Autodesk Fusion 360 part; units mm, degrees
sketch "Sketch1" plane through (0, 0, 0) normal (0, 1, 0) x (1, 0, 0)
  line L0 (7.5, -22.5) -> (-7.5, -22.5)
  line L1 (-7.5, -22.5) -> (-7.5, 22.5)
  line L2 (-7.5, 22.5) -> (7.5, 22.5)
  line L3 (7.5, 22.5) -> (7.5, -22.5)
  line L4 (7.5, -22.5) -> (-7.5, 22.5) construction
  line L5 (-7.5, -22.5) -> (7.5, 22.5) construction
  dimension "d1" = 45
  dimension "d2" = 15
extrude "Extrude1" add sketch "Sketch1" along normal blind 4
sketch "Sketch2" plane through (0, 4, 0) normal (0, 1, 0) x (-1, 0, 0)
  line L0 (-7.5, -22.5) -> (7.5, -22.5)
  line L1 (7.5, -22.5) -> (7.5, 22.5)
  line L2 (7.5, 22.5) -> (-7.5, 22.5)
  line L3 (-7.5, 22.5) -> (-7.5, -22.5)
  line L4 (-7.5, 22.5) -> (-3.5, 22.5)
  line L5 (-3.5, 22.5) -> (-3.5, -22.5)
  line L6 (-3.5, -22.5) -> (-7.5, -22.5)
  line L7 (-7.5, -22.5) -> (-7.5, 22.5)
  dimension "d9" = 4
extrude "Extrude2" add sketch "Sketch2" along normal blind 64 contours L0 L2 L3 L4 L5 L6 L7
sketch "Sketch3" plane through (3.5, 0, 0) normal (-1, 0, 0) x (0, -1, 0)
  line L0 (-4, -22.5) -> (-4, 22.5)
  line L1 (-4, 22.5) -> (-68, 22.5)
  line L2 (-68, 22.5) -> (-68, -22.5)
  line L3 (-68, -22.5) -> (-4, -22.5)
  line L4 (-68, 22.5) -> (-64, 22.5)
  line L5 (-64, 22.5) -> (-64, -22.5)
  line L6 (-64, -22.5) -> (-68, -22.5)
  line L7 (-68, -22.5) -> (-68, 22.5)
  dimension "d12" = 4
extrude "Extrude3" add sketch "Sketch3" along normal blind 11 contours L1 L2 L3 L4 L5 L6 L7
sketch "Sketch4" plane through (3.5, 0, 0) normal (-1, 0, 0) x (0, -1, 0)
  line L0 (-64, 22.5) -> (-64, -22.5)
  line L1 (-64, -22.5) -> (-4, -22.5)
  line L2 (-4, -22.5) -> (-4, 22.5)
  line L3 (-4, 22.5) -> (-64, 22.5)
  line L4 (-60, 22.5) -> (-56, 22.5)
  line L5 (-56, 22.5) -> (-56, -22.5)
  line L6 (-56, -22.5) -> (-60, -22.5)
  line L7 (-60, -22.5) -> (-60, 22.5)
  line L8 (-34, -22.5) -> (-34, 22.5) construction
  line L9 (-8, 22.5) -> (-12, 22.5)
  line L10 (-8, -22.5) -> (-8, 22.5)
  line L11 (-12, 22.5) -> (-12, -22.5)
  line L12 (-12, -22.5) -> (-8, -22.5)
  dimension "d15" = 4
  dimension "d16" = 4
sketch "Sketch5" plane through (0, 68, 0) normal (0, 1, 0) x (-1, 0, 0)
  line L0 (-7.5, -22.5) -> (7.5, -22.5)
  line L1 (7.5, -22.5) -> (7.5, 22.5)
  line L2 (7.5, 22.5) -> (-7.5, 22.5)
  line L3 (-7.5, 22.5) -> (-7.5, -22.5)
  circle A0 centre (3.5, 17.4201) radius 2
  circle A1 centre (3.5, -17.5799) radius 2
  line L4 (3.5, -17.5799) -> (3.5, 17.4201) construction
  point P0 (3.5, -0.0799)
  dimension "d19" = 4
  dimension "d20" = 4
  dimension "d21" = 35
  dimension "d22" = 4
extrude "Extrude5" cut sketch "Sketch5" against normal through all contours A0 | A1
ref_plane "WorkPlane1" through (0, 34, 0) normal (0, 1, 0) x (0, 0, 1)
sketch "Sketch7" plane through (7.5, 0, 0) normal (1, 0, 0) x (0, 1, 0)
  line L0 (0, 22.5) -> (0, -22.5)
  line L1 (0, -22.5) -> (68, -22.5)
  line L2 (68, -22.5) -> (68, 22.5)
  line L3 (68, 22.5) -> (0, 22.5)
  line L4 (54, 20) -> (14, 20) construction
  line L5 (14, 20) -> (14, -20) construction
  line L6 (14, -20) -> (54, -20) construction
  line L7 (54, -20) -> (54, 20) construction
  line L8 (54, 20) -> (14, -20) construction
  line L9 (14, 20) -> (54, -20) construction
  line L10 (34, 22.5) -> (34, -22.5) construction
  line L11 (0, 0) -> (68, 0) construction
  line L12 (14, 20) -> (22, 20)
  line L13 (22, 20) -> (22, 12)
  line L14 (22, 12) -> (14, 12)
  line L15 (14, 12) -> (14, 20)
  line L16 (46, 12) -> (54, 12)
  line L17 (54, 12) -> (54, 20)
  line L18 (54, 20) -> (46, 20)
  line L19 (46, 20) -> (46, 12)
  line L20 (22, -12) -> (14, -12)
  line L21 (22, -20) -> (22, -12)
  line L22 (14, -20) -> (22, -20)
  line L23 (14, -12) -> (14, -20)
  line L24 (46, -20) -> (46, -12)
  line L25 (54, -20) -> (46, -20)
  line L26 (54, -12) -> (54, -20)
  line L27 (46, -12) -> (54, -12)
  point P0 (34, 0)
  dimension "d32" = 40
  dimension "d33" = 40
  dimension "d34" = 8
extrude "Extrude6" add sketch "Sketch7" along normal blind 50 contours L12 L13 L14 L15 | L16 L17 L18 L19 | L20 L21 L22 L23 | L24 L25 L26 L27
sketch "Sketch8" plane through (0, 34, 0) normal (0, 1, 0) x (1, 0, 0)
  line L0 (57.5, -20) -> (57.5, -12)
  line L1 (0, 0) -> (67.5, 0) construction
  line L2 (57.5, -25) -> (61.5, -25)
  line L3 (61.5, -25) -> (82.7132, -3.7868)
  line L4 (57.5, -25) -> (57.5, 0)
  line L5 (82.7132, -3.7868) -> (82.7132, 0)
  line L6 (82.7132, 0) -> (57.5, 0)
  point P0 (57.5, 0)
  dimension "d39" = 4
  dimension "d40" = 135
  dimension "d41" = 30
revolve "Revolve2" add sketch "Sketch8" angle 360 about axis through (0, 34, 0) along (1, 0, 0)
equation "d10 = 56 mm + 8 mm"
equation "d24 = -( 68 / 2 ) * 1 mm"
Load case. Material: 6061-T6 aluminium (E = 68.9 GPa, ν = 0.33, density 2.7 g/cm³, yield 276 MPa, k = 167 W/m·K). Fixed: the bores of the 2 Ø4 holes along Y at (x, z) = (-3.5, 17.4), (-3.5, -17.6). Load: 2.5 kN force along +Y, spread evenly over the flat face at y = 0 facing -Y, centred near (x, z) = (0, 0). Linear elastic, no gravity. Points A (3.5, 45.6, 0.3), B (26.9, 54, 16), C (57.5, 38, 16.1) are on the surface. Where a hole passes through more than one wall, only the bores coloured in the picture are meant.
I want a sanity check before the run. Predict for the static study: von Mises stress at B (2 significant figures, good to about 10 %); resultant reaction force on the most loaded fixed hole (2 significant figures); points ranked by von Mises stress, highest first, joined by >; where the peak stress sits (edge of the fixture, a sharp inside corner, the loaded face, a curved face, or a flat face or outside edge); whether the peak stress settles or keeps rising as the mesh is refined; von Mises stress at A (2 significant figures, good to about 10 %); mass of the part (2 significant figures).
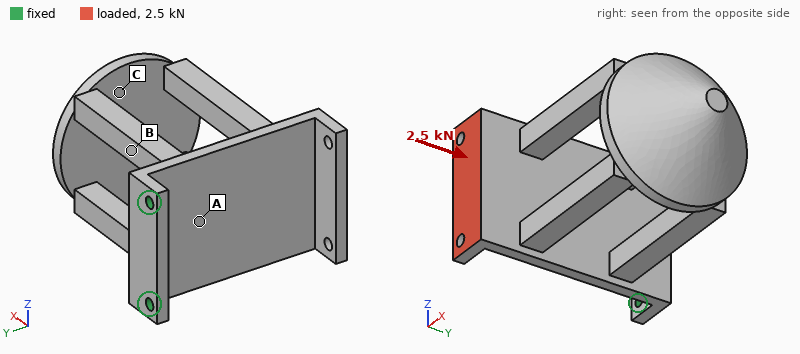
26 MPa
1.3 kN
A > B > C
edge of the fixture
keeps rising
52 MPa
140 g
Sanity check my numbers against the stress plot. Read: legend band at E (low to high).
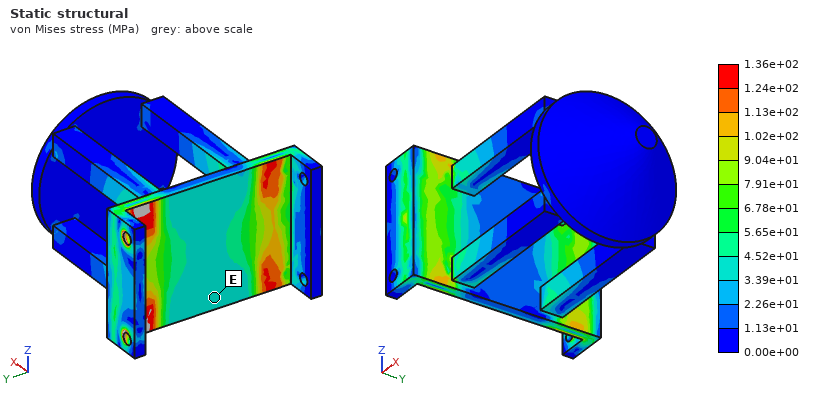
3.39e+01 to 4.52e+01 MPa
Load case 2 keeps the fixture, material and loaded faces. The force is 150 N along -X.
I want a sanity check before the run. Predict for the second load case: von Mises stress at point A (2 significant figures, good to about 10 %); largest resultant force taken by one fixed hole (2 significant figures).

27 MPa
110 N
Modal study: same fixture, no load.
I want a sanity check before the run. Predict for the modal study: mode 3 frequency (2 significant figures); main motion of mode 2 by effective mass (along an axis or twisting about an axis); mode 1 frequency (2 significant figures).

1600 Hz
along Z
190 Hz
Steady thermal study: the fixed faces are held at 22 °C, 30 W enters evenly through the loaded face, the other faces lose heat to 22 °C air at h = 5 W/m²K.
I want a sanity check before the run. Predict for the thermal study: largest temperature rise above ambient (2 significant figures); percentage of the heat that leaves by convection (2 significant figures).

68 K
11 %
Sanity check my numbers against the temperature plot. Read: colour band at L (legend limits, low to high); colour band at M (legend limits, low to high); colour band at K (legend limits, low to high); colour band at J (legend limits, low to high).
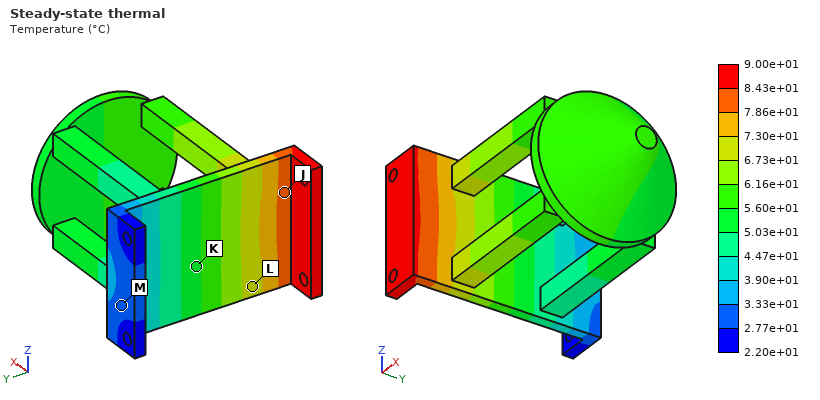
6.73e+01 to 7.30e+01 °C
2.77e+01 to 3.33e+01 °C
5.03e+01 to 5.60e+01 °C
7.86e+01 to 8.43e+01 °C
